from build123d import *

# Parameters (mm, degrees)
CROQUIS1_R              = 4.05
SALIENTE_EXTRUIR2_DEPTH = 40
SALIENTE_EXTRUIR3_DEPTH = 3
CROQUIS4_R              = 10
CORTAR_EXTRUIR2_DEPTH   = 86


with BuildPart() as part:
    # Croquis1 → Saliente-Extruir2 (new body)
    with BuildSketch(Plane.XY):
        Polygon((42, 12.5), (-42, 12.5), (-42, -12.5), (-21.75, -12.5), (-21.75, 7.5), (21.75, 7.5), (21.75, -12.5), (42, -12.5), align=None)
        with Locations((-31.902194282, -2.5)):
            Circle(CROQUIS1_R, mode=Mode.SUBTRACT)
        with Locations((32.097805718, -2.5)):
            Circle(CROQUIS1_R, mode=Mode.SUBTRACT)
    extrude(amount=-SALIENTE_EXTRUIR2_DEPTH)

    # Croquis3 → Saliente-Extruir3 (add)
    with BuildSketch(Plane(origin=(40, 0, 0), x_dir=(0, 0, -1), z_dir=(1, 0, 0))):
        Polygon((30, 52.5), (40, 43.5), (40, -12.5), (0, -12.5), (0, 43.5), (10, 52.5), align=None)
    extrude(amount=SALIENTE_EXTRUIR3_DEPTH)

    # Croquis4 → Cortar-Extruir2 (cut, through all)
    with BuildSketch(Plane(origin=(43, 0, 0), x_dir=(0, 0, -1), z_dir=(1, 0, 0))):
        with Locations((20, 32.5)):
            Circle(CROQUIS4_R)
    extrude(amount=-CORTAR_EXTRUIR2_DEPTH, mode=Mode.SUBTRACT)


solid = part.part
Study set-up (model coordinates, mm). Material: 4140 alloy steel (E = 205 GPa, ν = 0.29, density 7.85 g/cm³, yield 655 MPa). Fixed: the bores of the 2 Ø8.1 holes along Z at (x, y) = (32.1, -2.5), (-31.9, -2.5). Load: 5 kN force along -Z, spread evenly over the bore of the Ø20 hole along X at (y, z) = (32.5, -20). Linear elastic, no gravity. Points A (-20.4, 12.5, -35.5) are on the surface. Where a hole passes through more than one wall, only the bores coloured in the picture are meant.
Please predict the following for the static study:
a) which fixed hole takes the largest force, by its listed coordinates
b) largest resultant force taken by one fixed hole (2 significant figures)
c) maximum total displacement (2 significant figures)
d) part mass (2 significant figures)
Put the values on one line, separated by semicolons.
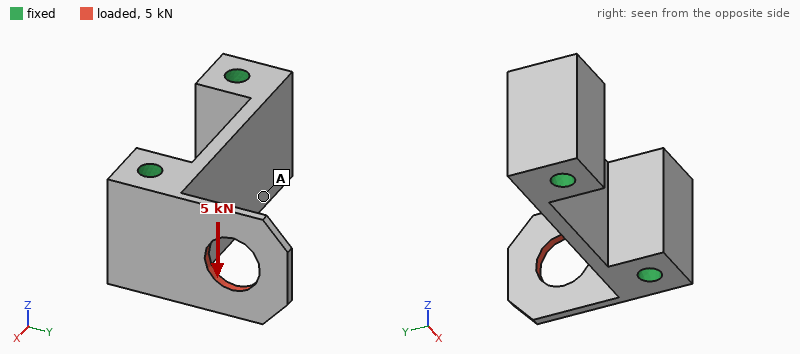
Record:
(32.1, -2.5); 4.9 kN; 69 µm; 390 g
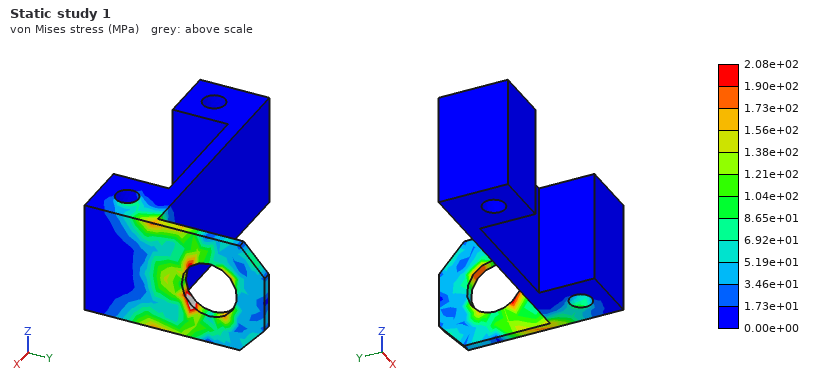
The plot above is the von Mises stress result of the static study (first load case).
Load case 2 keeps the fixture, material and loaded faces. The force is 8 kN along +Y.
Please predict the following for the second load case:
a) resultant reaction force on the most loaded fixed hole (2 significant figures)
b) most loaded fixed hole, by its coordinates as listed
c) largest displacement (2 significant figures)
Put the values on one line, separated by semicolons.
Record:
8.1 kN; (32.1, -2.5); 35 µm
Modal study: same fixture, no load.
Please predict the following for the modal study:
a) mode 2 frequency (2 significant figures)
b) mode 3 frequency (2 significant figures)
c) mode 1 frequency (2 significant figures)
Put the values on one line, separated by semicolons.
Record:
3800 Hz; 8300 Hz; 1500 Hz
